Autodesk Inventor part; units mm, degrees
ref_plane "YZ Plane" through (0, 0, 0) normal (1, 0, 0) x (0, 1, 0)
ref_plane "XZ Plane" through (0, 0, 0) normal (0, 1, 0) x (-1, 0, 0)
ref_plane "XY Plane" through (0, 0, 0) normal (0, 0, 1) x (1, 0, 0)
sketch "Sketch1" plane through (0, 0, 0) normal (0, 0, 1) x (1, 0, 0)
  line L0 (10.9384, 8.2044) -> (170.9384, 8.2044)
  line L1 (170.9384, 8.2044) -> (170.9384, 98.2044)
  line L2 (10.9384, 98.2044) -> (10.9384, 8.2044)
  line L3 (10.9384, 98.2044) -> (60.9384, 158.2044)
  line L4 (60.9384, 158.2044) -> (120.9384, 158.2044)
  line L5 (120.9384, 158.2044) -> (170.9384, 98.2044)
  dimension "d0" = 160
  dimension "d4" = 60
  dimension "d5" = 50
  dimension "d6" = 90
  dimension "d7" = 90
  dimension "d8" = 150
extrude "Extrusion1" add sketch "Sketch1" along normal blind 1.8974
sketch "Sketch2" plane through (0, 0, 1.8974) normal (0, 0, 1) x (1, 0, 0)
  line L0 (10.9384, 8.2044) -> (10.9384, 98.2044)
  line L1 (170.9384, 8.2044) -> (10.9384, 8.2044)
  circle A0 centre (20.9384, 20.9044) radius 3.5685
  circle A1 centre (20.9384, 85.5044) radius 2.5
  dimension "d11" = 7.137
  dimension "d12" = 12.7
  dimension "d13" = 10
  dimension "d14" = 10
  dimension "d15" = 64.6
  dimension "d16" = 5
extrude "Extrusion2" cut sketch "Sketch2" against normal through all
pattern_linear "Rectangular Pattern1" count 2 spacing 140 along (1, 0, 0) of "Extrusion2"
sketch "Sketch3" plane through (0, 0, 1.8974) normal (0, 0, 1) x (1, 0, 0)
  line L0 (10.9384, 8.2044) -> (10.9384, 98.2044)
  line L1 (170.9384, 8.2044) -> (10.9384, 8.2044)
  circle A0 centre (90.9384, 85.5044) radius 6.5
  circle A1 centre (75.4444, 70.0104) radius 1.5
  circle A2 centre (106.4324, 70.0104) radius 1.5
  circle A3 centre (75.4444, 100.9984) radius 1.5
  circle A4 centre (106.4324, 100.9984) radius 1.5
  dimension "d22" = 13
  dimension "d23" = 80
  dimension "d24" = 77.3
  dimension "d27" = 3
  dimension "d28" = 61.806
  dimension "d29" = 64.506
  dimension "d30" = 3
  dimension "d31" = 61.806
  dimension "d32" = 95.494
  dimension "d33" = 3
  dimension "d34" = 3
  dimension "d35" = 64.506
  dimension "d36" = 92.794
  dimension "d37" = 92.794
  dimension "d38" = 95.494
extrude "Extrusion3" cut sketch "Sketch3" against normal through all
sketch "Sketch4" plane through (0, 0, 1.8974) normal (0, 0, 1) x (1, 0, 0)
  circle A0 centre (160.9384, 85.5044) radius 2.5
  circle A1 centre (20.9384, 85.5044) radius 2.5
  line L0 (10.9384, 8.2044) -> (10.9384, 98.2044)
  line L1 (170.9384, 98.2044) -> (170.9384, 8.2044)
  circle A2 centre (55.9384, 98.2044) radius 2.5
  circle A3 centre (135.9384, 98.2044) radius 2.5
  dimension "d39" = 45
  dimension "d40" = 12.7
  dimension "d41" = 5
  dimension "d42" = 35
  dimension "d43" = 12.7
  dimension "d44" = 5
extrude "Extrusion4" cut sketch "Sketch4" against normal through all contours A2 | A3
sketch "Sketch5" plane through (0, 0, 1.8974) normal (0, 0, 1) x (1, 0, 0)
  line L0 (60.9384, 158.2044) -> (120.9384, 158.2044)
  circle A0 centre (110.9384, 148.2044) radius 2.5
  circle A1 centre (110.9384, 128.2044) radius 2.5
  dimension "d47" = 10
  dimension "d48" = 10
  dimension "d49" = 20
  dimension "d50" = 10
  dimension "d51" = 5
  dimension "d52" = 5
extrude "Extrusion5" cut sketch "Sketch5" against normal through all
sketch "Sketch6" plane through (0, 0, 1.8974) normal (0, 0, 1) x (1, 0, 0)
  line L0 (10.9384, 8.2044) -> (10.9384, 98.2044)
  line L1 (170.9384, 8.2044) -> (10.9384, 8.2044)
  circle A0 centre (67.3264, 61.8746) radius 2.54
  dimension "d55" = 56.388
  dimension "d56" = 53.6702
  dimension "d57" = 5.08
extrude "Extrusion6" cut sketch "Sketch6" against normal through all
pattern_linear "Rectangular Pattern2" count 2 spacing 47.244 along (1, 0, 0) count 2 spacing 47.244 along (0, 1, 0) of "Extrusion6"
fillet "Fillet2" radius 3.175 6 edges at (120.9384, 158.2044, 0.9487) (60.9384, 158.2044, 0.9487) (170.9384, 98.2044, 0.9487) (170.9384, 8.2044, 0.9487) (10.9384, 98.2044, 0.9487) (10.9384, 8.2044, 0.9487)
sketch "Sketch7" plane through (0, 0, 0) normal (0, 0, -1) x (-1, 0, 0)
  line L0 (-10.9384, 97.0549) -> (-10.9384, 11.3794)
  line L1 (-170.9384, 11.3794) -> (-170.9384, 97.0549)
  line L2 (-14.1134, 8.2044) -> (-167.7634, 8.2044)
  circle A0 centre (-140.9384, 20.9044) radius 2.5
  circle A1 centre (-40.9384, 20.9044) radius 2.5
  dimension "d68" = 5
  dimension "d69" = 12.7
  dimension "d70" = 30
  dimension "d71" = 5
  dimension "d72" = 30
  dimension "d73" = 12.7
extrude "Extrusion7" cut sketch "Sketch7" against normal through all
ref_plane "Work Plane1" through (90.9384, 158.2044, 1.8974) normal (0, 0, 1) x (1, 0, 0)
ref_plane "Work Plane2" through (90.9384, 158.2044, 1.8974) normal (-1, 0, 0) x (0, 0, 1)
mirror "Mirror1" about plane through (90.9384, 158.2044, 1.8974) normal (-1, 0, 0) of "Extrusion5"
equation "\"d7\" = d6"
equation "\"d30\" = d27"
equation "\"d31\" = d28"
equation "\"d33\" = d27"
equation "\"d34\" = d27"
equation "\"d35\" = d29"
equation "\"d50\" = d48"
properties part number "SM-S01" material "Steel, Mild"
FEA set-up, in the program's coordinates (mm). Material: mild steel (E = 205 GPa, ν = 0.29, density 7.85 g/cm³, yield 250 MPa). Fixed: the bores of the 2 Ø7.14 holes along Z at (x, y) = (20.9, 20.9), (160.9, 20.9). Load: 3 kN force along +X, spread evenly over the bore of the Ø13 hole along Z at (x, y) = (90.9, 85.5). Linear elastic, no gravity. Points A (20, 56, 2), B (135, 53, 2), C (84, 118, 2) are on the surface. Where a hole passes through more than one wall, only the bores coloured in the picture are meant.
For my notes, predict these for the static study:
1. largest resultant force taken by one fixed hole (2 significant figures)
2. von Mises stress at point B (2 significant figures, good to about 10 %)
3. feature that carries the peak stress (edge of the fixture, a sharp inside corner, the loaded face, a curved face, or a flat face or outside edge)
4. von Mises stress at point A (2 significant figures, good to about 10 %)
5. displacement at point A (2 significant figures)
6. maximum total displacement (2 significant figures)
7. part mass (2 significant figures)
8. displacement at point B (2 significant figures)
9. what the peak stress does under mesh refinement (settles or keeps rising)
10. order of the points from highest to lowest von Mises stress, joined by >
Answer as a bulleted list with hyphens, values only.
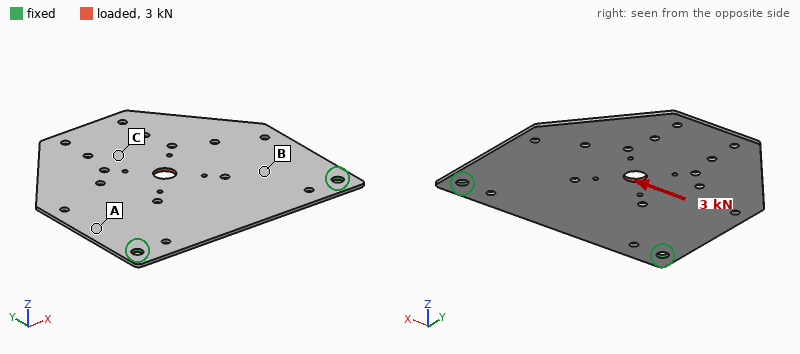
- 2.0 kN
- 22 MPa
- edge of the fixture
- 12 MPa
- 9.2 µm
- 18 µm
- 300 g
- 8.0 µm
- keeps rising
- B > A > C
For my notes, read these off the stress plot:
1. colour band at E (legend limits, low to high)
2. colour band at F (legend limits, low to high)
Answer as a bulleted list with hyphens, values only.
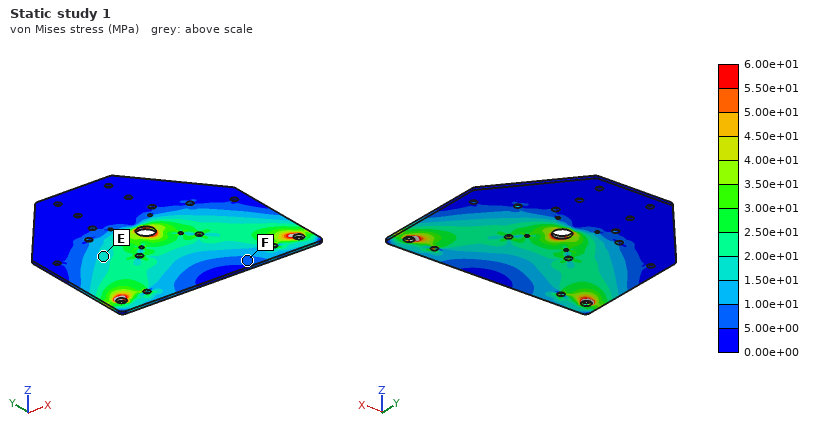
- 1.50e+01 to 2.00e+01 MPa
- 5.00e+00 to 1.00e+01 MPa
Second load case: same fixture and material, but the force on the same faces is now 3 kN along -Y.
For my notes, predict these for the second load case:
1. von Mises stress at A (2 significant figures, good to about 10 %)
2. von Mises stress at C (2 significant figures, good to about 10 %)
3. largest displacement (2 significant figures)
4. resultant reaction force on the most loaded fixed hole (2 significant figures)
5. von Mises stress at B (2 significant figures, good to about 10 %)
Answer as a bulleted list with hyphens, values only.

- 16 MPa
- 13 MPa
- 13 µm
- 1.6 kN
- 18 MPa
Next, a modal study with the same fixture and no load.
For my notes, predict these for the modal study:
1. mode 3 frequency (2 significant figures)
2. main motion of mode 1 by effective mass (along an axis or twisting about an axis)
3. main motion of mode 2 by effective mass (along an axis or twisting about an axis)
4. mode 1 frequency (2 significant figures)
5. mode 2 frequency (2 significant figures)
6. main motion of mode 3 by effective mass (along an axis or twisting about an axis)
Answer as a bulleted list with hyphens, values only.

- 440 Hz
- along Z
- twisting about Y
- 83 Hz
- 270 Hz
- along Z
